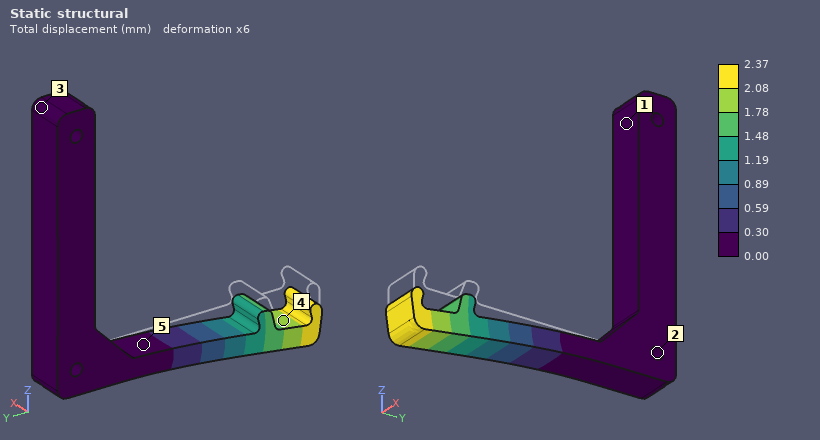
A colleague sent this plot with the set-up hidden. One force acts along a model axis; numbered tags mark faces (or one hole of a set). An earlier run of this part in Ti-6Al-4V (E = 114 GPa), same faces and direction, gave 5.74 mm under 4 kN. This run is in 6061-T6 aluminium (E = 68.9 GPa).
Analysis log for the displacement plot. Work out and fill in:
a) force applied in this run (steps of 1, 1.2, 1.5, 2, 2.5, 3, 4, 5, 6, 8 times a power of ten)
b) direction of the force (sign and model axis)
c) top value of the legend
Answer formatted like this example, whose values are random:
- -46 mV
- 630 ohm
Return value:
- 1 kN
- -Z
- 2.37 mm
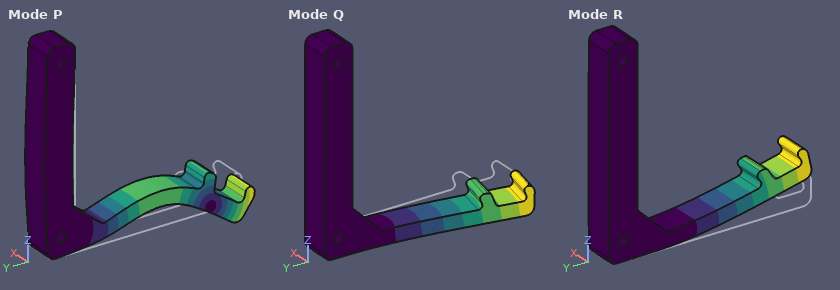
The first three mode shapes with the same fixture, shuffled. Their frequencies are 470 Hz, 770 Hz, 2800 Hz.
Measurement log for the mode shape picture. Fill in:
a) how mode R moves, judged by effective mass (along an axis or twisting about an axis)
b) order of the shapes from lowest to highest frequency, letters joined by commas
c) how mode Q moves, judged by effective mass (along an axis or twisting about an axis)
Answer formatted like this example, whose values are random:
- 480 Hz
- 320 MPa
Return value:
- along Z
- R, Q, P
- along X
